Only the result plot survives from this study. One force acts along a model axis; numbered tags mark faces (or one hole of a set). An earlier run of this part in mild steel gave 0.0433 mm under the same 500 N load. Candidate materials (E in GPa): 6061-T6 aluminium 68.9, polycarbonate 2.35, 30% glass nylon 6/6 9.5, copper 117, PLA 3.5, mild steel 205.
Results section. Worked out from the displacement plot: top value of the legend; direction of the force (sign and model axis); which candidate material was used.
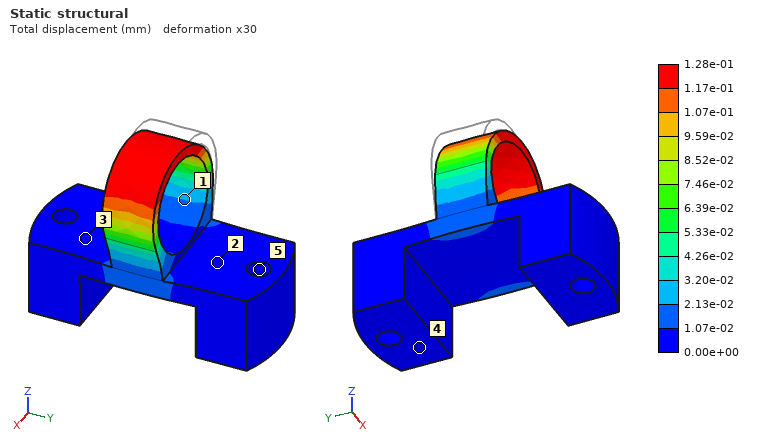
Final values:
1.28e-01 mm
+X
6061-T6 aluminium
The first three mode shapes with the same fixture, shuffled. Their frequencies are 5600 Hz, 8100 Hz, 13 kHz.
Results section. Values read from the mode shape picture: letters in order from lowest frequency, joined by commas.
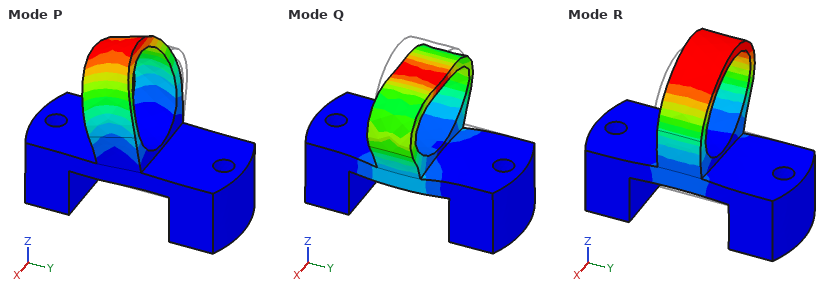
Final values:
R, P, Q
